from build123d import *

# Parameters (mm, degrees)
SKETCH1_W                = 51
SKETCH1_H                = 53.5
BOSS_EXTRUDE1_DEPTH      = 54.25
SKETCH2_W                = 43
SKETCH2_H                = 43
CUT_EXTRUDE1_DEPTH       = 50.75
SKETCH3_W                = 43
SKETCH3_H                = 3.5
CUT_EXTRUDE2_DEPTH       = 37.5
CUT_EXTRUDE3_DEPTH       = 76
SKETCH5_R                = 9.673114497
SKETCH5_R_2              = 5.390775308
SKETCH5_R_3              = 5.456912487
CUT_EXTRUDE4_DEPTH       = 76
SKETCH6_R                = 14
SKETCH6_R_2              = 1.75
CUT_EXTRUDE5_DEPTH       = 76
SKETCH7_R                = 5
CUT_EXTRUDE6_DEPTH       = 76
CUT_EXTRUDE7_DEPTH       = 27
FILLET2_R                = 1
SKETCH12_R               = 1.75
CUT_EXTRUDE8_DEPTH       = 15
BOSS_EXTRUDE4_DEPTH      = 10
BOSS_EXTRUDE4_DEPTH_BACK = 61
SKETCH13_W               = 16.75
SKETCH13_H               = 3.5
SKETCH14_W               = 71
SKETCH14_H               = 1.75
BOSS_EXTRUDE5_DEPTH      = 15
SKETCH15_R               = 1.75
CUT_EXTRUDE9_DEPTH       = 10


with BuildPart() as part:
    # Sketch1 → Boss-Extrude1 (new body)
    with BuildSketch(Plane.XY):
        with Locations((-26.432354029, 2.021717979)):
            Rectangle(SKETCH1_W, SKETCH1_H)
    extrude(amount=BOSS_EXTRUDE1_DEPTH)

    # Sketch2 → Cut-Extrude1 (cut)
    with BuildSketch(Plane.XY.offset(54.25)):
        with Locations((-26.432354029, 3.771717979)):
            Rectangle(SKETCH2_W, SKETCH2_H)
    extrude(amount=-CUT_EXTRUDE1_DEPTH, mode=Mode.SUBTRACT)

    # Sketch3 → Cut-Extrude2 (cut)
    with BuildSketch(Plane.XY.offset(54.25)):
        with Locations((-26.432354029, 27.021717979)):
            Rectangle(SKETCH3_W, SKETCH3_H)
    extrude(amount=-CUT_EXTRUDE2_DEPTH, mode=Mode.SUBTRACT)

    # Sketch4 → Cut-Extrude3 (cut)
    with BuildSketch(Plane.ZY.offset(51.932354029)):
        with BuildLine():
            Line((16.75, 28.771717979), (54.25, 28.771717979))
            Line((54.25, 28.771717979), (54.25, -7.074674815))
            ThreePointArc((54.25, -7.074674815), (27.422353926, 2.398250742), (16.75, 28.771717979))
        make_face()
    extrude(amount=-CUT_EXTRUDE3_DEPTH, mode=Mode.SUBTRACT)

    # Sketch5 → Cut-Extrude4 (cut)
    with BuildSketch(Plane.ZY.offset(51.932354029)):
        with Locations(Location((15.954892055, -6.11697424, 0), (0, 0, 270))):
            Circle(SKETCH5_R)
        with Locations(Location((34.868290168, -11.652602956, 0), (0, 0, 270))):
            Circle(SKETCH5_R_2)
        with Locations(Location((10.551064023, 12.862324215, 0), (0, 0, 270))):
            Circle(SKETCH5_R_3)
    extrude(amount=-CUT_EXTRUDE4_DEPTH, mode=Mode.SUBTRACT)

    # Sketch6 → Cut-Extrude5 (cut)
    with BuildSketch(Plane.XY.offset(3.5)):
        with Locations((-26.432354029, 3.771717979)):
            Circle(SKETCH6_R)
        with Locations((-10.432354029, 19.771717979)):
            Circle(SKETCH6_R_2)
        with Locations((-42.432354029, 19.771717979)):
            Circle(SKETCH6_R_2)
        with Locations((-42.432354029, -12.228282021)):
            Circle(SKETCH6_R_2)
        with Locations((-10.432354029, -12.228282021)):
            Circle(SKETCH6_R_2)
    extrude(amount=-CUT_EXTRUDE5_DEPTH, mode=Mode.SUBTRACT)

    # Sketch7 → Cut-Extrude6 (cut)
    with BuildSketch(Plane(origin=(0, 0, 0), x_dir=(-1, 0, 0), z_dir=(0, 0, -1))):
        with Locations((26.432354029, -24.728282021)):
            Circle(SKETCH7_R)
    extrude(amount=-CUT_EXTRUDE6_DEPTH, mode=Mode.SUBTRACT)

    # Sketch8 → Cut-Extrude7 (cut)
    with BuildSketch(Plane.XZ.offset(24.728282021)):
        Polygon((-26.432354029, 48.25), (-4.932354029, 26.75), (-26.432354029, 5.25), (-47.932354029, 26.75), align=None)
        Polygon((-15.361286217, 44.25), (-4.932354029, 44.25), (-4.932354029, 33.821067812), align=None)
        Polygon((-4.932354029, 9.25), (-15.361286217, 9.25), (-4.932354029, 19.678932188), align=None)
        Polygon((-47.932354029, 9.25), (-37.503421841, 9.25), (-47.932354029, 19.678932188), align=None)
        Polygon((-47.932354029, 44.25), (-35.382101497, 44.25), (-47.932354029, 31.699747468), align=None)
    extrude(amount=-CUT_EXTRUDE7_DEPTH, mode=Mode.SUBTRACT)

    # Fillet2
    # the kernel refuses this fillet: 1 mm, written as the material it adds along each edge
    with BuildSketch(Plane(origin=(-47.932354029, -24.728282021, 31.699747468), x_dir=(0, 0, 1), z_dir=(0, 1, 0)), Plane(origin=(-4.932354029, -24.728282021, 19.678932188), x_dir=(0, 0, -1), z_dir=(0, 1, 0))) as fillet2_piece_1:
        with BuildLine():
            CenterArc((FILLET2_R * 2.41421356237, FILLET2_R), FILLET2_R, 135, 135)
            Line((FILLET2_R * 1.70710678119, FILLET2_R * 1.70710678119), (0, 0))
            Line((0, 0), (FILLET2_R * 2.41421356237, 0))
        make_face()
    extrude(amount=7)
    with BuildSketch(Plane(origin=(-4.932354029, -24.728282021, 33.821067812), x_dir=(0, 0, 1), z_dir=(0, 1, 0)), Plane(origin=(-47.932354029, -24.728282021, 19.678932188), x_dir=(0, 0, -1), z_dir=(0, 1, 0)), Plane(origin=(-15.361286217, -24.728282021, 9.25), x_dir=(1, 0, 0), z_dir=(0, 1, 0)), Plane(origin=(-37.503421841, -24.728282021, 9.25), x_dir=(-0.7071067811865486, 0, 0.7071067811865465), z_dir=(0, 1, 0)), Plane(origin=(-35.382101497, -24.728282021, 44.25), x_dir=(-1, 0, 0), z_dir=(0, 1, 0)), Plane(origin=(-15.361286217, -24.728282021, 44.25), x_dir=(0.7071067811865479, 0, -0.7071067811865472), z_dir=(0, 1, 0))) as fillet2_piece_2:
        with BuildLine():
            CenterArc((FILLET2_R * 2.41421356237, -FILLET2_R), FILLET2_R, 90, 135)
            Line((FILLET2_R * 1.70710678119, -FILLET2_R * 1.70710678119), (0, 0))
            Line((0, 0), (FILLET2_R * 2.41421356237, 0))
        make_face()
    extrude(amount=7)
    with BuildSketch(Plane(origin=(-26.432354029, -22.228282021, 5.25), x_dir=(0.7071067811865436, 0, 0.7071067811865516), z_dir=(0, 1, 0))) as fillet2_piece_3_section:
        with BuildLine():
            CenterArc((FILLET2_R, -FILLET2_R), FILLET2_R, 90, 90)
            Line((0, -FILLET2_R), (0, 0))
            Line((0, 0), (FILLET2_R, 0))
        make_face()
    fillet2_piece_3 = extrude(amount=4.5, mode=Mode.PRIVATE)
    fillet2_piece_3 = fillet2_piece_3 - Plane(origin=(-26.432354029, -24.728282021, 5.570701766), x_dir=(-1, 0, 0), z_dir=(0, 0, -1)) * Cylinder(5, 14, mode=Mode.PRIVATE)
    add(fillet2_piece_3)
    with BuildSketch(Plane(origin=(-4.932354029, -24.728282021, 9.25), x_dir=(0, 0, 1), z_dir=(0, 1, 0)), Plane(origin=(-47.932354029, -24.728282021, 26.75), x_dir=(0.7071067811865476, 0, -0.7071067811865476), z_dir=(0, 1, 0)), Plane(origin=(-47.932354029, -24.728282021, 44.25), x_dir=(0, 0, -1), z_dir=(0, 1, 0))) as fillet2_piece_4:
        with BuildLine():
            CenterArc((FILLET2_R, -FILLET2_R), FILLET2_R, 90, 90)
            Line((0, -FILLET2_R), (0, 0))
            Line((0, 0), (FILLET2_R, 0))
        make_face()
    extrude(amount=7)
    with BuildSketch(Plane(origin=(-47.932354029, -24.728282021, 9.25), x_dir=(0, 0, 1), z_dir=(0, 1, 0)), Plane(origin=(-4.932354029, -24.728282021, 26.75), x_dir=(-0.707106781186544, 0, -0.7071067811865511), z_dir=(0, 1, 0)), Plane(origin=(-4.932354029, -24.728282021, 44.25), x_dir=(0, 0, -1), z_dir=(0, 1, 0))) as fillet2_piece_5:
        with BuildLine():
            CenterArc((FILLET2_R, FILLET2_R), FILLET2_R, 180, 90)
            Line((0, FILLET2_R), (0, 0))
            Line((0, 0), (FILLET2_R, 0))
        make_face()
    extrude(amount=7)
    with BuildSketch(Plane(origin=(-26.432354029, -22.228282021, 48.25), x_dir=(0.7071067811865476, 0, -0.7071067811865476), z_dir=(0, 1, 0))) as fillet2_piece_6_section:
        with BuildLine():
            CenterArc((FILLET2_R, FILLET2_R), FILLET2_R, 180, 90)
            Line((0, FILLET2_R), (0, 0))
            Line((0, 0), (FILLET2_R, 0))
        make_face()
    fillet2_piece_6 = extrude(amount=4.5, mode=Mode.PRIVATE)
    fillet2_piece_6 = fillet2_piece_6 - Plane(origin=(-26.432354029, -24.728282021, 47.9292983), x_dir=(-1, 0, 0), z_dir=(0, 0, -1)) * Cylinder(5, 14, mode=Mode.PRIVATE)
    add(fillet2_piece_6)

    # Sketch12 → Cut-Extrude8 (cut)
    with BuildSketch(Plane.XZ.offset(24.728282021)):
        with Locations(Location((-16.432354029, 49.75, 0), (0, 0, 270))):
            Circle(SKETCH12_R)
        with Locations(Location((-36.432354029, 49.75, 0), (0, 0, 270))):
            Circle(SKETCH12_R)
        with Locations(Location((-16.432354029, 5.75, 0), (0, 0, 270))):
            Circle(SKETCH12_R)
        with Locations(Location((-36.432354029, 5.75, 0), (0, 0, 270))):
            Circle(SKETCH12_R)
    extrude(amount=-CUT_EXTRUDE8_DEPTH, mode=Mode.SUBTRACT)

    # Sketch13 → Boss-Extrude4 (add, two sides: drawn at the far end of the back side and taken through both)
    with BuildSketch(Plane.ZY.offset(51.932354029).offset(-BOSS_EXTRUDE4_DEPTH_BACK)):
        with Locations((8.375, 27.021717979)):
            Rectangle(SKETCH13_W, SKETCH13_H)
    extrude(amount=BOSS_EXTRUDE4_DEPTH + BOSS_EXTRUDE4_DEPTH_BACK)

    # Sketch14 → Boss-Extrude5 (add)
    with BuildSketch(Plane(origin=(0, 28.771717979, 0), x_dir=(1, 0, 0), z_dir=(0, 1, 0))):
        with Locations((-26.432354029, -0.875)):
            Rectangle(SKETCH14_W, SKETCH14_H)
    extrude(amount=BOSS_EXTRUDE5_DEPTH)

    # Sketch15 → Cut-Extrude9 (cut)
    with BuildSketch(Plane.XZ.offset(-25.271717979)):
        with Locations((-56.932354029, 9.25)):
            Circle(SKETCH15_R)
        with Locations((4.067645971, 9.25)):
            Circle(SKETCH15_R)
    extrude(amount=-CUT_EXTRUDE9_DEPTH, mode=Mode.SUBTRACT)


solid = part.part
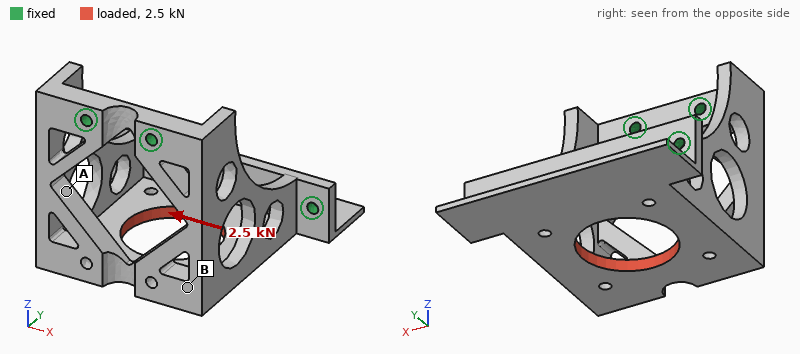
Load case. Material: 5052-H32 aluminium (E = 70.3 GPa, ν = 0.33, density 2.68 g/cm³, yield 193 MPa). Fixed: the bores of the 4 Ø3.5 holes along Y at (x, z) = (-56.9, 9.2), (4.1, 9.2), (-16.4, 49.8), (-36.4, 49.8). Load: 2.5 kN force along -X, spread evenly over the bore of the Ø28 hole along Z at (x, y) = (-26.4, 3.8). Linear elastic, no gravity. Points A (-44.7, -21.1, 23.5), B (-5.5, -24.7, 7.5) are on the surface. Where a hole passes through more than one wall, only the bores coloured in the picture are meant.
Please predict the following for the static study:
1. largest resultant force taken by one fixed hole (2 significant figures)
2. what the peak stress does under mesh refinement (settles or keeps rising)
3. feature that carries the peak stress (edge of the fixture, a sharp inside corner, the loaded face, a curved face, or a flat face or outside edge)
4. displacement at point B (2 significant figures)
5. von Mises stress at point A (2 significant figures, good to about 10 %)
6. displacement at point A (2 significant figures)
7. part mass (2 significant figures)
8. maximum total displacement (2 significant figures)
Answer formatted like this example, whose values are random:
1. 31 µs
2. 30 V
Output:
1. 1.3 kN
2. keeps rising
3. edge of the fixture
4. 45 µm
5. 16 MPa
6. 29 µm
7. 74 g
8. 52 µm
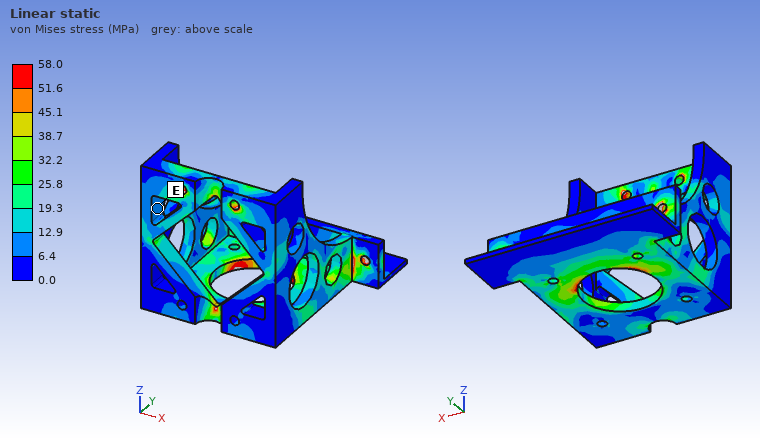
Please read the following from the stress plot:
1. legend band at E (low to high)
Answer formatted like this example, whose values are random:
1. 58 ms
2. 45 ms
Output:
1. 6.4 to 12.9 MPa
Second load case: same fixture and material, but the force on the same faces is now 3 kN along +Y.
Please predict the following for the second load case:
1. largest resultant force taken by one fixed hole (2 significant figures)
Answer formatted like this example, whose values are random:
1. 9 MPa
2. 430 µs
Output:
1. 1.4 kN
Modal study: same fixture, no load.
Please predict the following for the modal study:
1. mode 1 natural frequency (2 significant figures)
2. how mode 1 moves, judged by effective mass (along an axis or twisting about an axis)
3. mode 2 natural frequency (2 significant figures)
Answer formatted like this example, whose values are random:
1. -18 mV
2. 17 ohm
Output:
1. 5100 Hz
2. along Z
3. 5500 Hz
